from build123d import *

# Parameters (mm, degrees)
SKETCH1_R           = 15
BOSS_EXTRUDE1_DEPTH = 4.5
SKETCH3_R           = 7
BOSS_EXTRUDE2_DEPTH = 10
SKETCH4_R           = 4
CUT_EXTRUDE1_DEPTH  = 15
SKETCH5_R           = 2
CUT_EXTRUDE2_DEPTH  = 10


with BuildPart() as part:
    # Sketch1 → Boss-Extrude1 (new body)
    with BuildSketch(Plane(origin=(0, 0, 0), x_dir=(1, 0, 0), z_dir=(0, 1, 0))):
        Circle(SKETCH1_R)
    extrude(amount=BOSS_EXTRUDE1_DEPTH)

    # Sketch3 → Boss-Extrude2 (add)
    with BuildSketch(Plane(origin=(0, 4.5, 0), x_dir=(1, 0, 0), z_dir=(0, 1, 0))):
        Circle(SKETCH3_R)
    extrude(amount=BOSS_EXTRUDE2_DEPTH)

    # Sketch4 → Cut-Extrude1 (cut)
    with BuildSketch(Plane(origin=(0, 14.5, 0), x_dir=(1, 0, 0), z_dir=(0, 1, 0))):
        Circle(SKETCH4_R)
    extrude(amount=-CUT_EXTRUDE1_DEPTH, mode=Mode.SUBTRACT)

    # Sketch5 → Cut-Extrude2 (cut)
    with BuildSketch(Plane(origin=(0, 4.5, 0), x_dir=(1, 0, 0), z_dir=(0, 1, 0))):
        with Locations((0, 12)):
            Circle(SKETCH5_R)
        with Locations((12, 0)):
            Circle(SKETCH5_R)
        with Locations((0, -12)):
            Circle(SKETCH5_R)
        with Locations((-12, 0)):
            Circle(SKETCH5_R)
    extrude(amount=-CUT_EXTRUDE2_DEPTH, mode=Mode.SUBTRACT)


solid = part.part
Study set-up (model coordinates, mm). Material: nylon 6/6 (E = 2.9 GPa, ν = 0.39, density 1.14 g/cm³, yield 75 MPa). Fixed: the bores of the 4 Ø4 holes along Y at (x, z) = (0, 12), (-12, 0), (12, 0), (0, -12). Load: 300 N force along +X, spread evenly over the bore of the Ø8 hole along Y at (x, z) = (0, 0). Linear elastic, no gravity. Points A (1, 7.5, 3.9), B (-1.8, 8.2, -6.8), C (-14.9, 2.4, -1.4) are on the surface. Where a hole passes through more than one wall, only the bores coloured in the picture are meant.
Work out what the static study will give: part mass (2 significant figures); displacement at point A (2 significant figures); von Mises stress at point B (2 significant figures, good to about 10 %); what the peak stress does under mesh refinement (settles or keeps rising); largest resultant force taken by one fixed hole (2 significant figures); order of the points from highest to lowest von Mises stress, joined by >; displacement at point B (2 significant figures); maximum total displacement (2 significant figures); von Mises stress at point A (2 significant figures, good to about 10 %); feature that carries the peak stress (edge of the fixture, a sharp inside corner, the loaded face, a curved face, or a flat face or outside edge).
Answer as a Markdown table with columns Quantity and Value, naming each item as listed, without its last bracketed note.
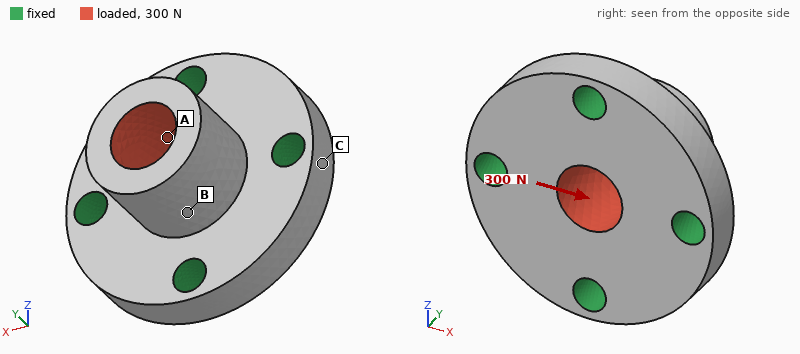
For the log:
| Quantity | Value |
|---|---|
| part mass | 4.3 g |
| displacement at point A | 20 µm |
| von Mises stress at point B | 2.7 MPa |
| what the peak stress does under mesh refinement | keeps rising |
| largest resultant force taken by one fixed hole | 120 N |
| order of the points from highest to lowest von Mises stress, joined by > | A > B > C |
| displacement at point B | 22 µm |
| maximum total displacement | 47 µm |
| von Mises stress at point A | 5.1 MPa |
| feature that carries the peak stress | edge of the fixture |
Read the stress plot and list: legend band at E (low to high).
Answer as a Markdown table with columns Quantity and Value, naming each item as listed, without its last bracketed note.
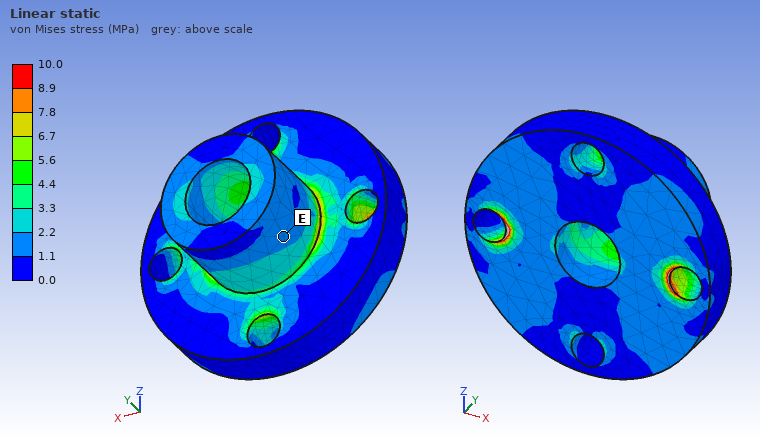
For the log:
| Quantity | Value |
|---|---|
| legend band at E | 1.1 to 2.2 MPa |
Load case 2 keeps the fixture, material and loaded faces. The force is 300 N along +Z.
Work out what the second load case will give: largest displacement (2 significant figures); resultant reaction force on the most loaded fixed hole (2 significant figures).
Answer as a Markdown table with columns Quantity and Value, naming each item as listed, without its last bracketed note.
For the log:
| Quantity | Value |
|---|---|
| largest displacement | 47 µm |
| resultant reaction force on the most loaded fixed hole | 120 N |
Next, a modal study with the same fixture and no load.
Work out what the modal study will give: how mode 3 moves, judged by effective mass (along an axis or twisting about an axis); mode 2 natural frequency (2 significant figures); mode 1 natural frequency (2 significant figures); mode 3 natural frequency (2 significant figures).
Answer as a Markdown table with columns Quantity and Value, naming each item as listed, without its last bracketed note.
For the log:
| Quantity | Value |
|---|---|
| how mode 3 moves, judged by effective mass | along Y |
| mode 2 natural frequency | 11 kHz |
| mode 1 natural frequency | 11 kHz |
| mode 3 natural frequency | 15 kHz |
